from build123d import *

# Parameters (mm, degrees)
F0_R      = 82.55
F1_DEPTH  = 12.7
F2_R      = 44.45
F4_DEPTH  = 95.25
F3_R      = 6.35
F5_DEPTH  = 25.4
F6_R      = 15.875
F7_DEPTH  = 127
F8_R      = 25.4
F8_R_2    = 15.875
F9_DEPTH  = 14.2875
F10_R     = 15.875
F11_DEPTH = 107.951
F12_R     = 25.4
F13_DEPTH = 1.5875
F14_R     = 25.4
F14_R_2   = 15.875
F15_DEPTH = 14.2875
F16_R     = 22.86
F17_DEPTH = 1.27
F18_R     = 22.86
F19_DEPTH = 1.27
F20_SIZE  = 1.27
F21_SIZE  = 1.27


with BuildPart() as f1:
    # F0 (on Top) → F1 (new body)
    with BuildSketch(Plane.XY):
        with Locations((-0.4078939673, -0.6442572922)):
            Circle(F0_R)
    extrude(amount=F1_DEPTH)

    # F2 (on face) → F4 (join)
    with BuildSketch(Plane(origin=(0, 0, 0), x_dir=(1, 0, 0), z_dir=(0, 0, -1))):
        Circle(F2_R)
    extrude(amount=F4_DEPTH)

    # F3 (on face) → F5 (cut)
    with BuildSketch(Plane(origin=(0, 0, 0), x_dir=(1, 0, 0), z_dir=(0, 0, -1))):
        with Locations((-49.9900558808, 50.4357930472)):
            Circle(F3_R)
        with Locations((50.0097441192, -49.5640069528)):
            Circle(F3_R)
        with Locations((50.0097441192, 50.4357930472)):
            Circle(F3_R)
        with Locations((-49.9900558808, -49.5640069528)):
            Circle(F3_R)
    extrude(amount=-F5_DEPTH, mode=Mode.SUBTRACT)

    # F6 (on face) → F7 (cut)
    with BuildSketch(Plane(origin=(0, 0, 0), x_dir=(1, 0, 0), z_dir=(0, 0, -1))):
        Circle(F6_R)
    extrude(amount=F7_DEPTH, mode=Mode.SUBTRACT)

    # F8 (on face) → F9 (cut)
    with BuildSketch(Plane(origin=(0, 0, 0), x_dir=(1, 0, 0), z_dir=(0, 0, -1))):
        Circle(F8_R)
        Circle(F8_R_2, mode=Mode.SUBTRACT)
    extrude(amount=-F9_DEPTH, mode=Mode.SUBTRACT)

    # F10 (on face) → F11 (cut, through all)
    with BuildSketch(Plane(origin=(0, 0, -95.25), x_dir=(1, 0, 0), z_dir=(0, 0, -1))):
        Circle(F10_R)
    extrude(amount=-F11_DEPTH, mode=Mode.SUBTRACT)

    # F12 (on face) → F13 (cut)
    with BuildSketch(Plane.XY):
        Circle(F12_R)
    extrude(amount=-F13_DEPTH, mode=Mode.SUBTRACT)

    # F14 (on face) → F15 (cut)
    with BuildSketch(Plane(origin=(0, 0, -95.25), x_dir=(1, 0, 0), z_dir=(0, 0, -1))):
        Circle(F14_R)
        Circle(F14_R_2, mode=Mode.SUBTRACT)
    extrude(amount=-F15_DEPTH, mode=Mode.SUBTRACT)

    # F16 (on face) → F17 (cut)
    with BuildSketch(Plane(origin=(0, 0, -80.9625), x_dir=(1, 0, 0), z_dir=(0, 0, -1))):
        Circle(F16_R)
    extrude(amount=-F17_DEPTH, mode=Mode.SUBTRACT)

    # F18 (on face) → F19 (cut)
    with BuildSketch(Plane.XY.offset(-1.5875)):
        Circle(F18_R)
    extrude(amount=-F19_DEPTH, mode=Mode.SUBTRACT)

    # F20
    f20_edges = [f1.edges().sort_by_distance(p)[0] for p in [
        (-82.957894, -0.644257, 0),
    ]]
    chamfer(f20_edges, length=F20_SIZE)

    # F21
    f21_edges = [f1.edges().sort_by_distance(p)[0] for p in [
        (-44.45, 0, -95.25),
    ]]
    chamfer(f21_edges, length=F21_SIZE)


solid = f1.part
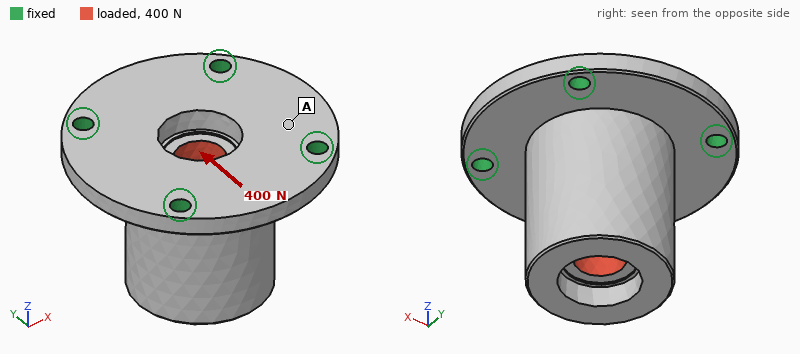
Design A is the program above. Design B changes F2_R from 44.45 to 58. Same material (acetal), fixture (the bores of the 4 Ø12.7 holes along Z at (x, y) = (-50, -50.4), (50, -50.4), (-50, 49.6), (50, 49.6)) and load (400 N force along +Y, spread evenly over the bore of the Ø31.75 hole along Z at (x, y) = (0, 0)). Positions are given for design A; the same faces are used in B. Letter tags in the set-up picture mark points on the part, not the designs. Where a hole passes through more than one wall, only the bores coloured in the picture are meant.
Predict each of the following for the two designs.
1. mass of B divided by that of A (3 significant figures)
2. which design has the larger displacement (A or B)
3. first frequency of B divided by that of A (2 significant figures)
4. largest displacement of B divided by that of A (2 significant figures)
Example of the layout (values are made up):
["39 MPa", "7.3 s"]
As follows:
["1.57", "A", "1.2", "0.35"]
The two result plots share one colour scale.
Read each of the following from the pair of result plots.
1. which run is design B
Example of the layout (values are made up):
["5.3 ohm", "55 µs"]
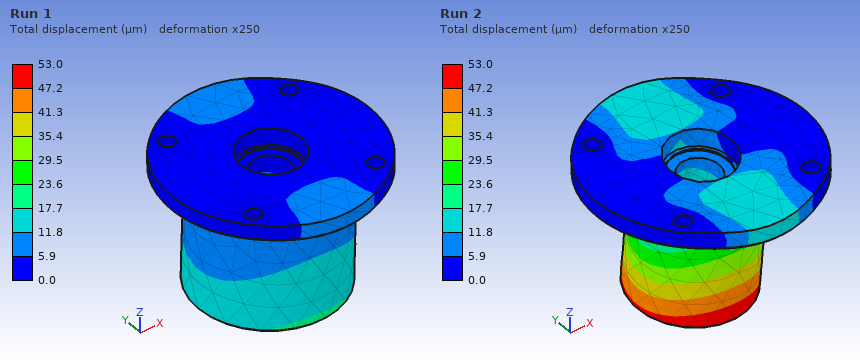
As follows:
["Run 1"]
